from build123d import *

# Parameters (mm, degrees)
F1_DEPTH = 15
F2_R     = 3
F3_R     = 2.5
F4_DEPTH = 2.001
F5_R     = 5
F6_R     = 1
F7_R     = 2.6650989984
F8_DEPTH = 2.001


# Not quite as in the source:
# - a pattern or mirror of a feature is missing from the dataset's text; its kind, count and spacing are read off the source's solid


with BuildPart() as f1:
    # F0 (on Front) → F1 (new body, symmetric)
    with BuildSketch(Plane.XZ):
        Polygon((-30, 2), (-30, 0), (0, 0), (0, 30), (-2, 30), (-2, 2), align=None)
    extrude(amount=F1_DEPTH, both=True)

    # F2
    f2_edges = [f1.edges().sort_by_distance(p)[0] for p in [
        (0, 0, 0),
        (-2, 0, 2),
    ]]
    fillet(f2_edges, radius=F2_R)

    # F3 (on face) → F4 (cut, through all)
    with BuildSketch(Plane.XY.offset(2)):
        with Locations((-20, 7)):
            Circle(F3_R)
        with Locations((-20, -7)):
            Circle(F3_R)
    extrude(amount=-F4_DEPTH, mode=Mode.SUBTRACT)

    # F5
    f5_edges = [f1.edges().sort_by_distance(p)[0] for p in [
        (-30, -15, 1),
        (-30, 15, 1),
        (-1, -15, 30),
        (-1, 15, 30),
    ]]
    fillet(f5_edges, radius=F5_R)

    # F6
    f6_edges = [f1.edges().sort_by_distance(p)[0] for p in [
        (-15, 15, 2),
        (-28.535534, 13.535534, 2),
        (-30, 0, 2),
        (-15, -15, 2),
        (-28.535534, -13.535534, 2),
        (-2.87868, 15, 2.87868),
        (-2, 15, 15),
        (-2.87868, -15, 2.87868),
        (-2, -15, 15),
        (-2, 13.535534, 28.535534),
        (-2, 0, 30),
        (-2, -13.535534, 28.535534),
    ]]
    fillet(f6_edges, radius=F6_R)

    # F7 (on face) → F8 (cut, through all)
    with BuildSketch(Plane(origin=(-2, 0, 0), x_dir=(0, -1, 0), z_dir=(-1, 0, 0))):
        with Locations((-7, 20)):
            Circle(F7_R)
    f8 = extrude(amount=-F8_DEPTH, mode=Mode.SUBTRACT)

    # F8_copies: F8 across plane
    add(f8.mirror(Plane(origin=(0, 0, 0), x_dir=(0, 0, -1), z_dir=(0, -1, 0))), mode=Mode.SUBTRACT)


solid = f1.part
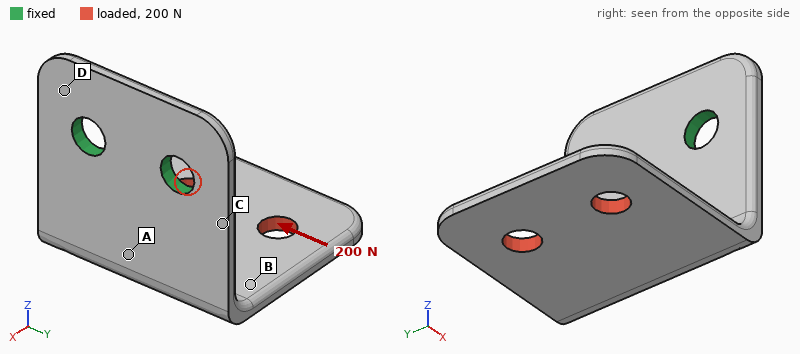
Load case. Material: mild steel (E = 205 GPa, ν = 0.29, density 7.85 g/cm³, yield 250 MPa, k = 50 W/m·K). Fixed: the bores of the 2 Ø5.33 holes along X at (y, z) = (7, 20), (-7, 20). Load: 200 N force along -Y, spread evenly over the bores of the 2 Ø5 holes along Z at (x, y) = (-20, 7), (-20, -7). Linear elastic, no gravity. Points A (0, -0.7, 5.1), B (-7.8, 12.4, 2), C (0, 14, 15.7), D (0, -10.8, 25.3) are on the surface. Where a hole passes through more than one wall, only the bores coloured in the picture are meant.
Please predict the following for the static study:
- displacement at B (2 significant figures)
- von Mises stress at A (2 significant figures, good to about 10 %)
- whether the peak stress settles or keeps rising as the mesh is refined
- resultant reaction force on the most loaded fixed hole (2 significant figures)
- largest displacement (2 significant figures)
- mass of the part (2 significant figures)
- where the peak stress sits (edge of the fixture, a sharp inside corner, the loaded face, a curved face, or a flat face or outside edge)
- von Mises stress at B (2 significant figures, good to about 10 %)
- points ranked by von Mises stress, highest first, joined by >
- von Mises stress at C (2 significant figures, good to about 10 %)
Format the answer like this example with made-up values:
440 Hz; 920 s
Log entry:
0.067 mm; 81 MPa; keeps rising; 290 N; 0.15 mm; 25 g; edge of the fixture; 56 MPa; C > A > B > D; 110 MPa
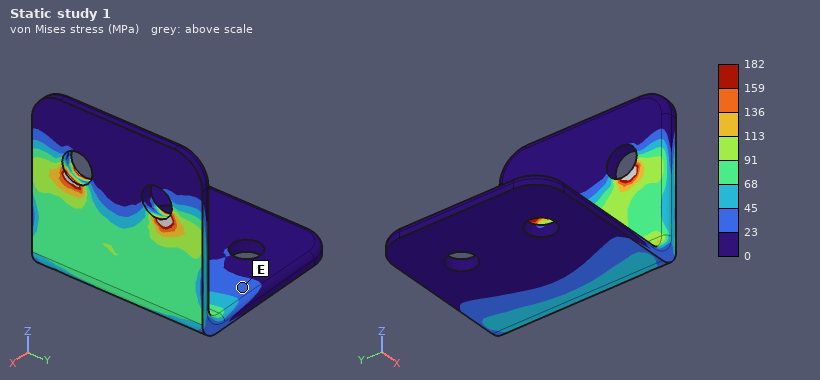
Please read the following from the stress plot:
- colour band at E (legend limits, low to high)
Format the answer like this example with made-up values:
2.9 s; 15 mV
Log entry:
23 to 45 MPa
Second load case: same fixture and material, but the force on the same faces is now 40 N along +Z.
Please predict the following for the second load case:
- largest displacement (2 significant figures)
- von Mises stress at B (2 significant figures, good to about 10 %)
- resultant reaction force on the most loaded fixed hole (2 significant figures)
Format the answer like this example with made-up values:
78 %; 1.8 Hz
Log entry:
0.11 mm; 23 MPa; 21 N
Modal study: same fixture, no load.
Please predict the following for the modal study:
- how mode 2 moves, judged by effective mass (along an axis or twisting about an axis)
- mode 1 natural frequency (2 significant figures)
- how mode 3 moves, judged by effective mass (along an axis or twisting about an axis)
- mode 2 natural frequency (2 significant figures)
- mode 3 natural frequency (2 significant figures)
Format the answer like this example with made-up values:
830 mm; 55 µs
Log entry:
along Y; 1100 Hz; along X; 2100 Hz; 3500 Hz
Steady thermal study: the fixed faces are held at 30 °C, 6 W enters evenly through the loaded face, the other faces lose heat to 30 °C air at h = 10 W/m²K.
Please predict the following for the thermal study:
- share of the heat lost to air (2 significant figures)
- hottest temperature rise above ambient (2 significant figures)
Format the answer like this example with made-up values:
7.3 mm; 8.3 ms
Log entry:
17 %; 66 K
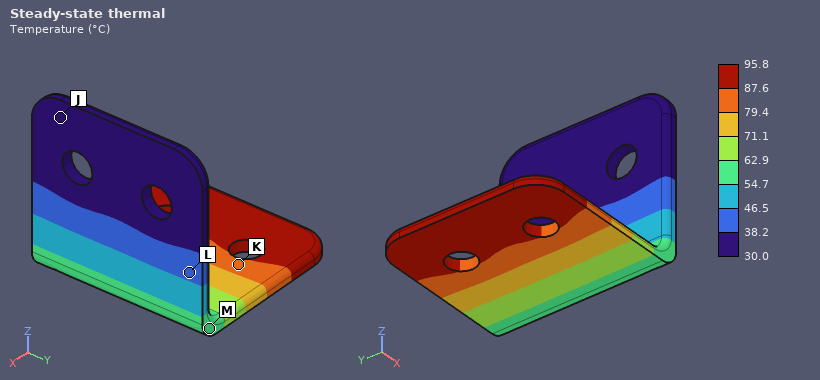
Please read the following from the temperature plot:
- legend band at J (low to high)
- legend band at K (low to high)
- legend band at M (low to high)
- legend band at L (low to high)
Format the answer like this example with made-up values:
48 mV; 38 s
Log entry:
30.0 to 38.2 °C; 79.4 to 87.6 °C; 54.7 to 62.9 °C; 38.2 to 46.5 °C
